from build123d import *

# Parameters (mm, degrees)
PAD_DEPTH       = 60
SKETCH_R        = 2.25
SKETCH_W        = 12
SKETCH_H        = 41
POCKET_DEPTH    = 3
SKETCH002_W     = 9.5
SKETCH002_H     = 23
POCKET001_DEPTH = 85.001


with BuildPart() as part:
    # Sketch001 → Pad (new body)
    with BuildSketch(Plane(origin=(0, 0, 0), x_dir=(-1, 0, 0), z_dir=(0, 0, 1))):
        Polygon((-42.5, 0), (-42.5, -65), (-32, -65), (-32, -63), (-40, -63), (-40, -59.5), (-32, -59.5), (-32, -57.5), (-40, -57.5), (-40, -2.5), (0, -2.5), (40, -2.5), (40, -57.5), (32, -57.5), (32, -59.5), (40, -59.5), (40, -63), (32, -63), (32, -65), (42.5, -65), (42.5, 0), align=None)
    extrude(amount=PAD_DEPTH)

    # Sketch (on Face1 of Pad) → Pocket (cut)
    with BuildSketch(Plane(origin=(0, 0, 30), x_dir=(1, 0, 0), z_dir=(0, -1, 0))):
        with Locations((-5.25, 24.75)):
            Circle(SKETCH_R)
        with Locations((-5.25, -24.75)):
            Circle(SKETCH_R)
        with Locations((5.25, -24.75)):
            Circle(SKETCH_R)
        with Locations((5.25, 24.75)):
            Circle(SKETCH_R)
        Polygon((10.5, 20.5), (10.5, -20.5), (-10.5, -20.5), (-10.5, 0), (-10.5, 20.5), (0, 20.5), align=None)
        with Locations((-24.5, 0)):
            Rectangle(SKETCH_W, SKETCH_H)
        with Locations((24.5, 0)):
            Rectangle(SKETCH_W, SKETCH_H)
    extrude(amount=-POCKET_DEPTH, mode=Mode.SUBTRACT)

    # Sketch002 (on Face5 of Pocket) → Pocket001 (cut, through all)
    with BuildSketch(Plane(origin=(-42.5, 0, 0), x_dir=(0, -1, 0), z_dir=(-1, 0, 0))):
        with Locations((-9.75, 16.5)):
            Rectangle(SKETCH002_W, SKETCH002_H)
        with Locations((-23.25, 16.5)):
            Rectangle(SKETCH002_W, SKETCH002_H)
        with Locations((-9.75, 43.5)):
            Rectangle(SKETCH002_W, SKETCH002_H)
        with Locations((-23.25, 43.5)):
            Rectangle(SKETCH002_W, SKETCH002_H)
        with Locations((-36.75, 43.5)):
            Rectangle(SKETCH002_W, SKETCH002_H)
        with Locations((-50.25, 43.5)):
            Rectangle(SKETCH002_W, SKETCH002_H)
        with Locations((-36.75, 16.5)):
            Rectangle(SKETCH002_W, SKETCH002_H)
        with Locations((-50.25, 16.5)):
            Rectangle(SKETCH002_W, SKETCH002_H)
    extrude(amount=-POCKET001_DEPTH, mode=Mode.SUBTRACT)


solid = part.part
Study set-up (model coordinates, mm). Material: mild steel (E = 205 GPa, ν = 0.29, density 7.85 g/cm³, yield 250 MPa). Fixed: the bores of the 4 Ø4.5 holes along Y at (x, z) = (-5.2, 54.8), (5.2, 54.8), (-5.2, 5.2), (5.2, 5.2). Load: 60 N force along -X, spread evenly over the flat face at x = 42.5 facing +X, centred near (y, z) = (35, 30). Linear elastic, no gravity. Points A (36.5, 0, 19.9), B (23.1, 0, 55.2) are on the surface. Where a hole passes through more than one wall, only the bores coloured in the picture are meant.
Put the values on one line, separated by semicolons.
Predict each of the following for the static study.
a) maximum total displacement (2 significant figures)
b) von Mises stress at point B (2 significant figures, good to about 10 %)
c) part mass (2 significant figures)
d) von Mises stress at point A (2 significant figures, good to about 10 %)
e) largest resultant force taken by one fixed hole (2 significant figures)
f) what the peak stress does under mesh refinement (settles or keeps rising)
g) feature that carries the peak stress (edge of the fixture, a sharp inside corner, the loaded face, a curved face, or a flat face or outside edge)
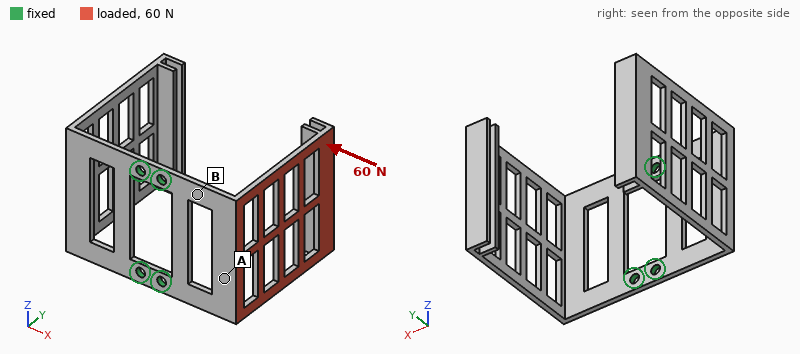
1.3 mm; 99 MPa; 170 g; 17 MPa; 28 N; keeps rising; edge of the fixture
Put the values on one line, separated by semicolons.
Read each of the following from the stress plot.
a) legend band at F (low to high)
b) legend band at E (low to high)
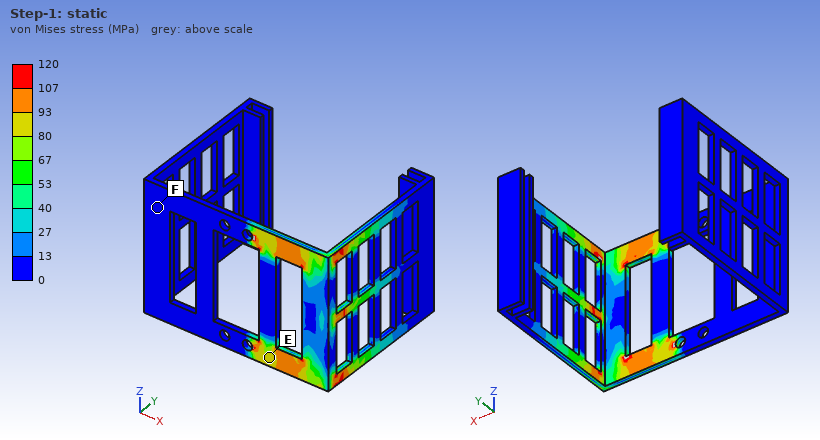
0 to 13 MPa; 80 to 93 MPa
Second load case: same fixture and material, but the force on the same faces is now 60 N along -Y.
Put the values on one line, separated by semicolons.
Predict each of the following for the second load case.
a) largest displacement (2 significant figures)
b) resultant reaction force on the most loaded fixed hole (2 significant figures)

0.49 mm; 32 N
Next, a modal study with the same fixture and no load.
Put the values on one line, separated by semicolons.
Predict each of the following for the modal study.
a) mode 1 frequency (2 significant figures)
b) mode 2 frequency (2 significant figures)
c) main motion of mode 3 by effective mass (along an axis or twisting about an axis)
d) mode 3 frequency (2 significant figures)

140 Hz; 140 Hz; along Z; 390 Hz
